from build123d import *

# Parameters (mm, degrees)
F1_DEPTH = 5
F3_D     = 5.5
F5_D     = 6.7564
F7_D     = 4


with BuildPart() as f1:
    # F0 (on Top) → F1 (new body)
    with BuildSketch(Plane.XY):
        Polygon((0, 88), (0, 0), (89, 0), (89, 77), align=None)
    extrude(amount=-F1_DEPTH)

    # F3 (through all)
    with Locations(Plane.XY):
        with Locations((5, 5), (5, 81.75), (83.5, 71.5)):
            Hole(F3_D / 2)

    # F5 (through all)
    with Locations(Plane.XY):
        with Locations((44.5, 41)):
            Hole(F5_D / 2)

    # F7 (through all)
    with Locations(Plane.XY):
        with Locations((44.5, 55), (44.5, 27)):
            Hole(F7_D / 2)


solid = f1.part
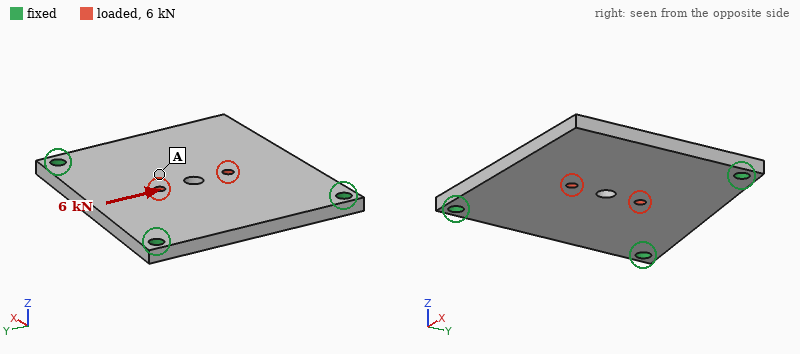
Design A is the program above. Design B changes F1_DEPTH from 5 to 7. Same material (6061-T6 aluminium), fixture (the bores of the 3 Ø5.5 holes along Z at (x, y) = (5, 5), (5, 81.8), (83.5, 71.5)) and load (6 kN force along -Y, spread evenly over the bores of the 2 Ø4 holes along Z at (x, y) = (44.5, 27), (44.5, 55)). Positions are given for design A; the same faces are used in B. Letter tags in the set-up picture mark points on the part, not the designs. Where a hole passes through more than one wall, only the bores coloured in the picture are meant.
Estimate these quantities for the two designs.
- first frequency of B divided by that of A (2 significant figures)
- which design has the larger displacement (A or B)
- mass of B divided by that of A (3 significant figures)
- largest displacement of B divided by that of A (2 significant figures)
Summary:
1.4
A
1.40
0.71
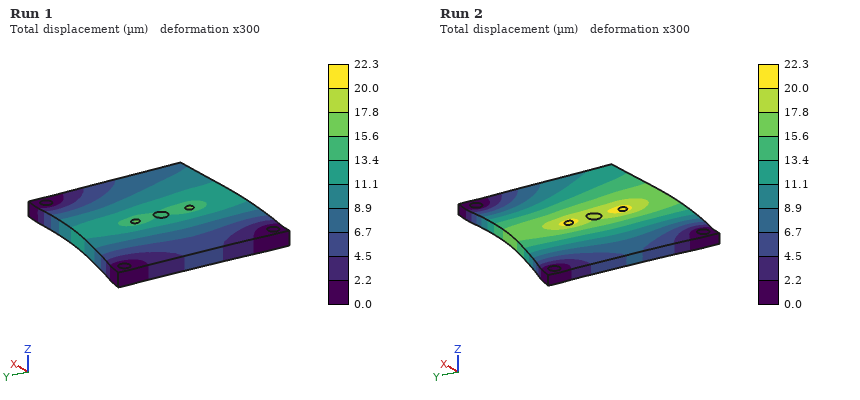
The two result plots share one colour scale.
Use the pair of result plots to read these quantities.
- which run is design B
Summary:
Run 1
